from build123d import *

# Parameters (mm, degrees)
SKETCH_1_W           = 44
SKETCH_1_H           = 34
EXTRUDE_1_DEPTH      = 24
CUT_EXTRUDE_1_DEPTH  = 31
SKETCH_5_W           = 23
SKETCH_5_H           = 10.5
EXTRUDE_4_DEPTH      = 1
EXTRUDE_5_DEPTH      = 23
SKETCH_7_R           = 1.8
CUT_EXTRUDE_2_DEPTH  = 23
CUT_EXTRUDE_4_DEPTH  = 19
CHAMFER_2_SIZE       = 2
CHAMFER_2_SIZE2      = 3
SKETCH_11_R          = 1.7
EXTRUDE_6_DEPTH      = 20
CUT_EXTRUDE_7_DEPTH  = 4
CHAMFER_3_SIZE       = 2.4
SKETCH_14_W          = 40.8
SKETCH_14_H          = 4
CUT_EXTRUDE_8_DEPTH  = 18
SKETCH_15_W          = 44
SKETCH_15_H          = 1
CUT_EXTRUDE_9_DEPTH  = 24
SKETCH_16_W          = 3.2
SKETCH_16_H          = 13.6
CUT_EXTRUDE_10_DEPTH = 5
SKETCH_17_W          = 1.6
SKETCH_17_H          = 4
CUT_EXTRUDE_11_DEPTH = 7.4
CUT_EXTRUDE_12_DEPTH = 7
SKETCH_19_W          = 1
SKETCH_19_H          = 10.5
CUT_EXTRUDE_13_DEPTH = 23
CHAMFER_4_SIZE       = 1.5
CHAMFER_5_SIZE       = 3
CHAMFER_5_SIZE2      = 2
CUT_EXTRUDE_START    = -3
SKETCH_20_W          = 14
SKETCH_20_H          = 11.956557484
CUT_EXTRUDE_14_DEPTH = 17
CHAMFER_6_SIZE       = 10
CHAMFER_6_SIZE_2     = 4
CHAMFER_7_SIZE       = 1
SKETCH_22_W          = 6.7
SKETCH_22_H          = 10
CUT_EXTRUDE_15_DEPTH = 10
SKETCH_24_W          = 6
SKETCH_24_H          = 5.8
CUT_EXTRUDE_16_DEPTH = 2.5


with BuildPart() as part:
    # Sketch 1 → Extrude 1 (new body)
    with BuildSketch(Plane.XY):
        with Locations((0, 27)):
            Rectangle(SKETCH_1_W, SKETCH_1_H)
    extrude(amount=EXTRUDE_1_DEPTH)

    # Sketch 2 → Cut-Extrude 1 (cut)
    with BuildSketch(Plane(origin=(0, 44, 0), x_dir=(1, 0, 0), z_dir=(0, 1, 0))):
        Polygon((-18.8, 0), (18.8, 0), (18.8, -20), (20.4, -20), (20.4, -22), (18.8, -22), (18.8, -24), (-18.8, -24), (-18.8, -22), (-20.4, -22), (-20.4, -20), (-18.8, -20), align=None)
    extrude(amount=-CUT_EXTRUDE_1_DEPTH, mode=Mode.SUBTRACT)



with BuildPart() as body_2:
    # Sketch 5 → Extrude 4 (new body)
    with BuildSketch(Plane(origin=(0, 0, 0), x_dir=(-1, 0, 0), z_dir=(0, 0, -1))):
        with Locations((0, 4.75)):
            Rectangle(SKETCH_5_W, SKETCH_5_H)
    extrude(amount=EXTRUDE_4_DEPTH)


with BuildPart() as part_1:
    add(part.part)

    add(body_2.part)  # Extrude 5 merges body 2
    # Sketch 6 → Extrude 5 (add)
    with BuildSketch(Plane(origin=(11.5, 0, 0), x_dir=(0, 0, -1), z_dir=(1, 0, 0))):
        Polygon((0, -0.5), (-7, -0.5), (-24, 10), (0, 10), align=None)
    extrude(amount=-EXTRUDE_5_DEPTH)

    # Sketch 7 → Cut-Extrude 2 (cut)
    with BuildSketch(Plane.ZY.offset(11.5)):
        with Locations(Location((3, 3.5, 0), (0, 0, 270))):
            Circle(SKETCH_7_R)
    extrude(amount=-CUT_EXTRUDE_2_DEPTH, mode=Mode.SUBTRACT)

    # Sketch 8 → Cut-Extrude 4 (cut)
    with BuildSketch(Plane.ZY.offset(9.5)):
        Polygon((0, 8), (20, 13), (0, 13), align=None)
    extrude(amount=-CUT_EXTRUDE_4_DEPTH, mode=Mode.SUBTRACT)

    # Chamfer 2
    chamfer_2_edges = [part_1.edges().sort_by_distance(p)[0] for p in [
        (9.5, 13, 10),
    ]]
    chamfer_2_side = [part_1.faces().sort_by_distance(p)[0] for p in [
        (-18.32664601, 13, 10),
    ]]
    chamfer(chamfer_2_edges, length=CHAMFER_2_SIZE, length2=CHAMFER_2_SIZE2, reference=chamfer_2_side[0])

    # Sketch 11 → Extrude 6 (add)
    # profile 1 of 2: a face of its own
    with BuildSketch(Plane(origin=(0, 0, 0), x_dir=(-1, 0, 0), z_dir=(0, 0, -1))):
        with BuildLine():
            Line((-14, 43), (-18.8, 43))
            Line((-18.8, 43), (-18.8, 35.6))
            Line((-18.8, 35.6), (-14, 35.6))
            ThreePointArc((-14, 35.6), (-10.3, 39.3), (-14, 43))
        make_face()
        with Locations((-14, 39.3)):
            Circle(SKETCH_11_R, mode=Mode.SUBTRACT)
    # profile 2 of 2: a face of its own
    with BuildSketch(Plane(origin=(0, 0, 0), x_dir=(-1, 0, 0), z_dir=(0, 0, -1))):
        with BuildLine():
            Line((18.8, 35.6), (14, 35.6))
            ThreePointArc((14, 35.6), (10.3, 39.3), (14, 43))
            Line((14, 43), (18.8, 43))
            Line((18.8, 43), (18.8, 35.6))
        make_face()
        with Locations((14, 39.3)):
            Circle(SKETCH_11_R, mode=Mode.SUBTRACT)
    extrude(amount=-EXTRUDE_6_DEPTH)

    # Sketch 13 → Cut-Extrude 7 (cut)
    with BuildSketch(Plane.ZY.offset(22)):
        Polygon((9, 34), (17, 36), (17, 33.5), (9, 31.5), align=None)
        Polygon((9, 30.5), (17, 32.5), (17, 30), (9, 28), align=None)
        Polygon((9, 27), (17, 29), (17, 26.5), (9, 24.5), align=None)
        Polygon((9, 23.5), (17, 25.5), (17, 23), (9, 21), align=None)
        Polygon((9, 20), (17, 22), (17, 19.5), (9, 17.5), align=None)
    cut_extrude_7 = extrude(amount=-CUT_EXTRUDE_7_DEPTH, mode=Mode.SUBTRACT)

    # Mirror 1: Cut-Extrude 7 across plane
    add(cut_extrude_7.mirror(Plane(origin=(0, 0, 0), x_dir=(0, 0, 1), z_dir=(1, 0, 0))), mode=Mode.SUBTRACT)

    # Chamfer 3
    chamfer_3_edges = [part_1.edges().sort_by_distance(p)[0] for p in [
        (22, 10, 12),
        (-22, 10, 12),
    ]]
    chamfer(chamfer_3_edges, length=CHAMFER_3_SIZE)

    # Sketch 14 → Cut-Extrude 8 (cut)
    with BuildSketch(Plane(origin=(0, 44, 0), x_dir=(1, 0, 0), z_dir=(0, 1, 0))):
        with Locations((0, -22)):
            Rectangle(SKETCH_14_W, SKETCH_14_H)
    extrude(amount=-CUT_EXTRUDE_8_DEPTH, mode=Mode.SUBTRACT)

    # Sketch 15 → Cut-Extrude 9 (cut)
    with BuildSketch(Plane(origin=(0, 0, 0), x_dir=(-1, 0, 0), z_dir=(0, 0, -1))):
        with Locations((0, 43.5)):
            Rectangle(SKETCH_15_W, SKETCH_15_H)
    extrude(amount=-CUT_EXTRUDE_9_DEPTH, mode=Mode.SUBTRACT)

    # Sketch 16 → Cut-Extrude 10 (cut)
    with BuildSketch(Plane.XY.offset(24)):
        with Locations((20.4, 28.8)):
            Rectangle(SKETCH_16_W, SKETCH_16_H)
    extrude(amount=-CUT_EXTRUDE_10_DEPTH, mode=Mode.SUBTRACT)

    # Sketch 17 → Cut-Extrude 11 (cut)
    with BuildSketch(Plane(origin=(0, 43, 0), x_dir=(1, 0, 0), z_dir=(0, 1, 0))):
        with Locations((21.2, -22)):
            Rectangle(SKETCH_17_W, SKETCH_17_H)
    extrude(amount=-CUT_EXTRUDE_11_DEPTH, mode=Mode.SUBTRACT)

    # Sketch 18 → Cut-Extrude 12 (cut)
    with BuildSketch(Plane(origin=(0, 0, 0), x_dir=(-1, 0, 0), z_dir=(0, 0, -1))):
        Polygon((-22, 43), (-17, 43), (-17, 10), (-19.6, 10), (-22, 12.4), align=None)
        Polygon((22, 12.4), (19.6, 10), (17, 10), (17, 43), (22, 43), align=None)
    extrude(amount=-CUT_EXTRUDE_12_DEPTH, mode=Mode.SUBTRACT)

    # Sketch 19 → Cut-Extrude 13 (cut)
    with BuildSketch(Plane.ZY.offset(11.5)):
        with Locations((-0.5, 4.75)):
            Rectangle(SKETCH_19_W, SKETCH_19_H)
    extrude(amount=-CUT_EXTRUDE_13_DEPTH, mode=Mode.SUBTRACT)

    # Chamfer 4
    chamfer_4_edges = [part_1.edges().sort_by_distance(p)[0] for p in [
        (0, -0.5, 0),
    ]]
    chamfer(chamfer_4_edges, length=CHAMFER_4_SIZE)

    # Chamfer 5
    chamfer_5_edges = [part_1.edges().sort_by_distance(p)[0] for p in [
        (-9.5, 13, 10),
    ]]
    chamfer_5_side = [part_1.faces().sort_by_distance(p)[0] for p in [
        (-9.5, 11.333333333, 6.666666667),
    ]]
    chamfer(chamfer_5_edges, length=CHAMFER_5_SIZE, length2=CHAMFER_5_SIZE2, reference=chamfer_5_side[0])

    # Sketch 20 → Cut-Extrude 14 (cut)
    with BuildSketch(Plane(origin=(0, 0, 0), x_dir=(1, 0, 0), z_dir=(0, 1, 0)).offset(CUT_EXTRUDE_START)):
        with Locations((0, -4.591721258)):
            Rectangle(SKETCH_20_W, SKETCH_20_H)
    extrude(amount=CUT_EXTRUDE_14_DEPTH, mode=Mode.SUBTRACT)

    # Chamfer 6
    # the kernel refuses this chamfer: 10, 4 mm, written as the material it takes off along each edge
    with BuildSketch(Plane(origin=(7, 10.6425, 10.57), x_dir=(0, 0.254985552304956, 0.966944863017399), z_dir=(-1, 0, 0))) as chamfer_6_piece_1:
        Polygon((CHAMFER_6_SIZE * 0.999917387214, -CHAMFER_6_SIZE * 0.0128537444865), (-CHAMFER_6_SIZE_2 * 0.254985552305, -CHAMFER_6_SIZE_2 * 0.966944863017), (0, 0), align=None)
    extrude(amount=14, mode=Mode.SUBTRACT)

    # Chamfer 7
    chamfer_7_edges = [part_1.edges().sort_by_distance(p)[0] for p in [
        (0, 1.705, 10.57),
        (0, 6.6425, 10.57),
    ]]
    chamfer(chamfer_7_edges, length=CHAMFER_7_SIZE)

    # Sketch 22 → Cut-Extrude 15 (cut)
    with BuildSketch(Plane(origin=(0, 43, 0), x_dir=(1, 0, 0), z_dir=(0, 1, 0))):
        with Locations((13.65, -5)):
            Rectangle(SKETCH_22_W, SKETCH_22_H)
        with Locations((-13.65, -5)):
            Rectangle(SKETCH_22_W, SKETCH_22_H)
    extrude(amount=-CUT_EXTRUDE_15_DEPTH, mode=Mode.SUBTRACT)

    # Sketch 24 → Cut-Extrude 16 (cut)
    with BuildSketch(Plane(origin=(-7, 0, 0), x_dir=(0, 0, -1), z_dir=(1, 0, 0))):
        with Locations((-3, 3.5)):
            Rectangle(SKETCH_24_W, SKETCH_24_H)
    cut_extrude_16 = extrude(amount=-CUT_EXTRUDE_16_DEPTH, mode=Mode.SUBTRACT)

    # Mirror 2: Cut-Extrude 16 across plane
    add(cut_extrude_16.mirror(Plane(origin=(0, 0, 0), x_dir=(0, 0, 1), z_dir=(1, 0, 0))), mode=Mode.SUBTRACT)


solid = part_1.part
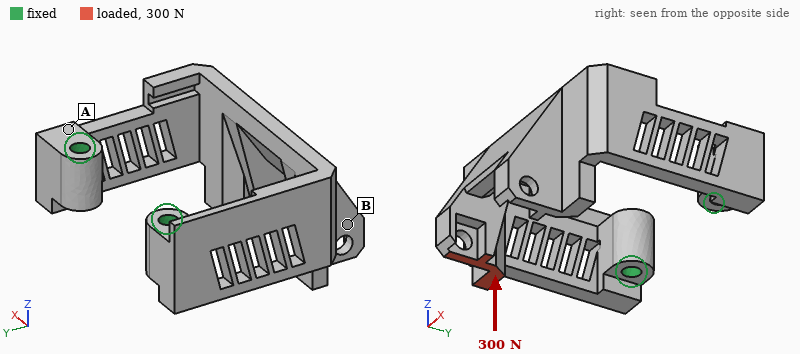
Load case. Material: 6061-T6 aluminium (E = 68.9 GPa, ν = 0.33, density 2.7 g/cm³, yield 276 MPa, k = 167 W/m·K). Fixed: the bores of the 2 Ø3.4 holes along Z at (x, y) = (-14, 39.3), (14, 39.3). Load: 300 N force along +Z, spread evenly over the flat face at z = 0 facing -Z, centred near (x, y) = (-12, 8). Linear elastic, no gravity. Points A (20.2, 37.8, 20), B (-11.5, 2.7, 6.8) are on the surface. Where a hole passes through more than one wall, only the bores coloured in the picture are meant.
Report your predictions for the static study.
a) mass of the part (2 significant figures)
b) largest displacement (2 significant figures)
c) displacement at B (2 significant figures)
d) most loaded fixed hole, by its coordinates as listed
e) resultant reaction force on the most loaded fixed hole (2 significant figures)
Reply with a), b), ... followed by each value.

a) 18 g
b) 0.20 mm
c) 0.18 mm
d) (-14, 39.3)
e) 230 N
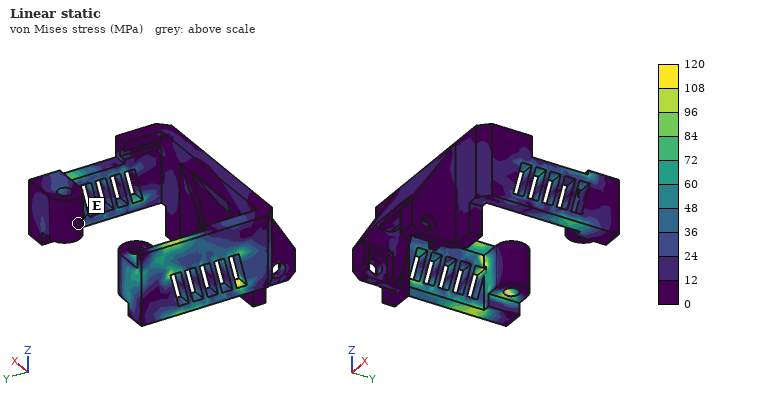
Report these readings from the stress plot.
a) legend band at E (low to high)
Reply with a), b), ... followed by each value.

a) 0 to 12 MPa
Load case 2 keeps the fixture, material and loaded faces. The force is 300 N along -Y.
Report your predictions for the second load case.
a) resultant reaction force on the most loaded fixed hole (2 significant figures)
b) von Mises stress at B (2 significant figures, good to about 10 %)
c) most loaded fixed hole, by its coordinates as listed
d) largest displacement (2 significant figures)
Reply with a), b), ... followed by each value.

a) 240 N
b) 12 MPa
c) (-14, 39.3)
d) 0.20 mm
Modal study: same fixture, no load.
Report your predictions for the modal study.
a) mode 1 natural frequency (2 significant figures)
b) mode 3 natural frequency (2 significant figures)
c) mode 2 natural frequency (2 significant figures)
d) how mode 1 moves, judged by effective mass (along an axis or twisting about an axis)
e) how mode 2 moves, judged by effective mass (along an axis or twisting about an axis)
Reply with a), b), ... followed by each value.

a) 1700 Hz
b) 3700 Hz
c) 2000 Hz
d) along X
e) along Z
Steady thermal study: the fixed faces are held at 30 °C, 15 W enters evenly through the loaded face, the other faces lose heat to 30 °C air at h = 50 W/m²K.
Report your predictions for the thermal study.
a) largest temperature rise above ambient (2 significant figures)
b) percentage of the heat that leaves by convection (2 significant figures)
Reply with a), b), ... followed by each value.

a) 64 K
b) 46 %
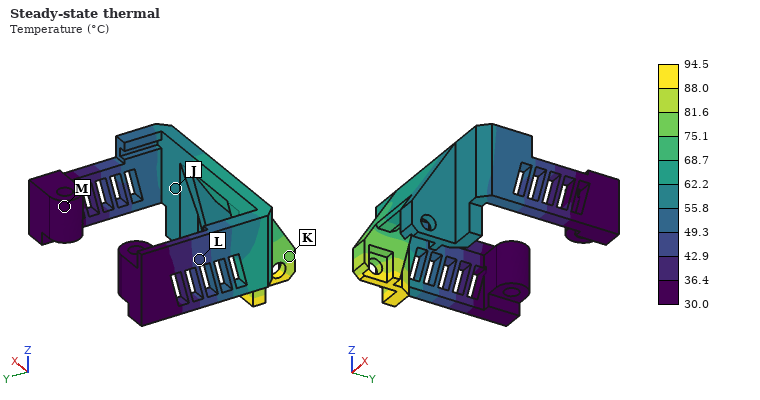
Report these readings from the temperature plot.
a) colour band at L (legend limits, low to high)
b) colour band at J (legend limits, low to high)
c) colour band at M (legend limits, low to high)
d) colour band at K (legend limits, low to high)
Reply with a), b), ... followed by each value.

a) 42.9 to 49.3 °C
b) 55.8 to 62.2 °C
c) 30.0 to 36.4 °C
d) 75.1 to 81.6 °C
